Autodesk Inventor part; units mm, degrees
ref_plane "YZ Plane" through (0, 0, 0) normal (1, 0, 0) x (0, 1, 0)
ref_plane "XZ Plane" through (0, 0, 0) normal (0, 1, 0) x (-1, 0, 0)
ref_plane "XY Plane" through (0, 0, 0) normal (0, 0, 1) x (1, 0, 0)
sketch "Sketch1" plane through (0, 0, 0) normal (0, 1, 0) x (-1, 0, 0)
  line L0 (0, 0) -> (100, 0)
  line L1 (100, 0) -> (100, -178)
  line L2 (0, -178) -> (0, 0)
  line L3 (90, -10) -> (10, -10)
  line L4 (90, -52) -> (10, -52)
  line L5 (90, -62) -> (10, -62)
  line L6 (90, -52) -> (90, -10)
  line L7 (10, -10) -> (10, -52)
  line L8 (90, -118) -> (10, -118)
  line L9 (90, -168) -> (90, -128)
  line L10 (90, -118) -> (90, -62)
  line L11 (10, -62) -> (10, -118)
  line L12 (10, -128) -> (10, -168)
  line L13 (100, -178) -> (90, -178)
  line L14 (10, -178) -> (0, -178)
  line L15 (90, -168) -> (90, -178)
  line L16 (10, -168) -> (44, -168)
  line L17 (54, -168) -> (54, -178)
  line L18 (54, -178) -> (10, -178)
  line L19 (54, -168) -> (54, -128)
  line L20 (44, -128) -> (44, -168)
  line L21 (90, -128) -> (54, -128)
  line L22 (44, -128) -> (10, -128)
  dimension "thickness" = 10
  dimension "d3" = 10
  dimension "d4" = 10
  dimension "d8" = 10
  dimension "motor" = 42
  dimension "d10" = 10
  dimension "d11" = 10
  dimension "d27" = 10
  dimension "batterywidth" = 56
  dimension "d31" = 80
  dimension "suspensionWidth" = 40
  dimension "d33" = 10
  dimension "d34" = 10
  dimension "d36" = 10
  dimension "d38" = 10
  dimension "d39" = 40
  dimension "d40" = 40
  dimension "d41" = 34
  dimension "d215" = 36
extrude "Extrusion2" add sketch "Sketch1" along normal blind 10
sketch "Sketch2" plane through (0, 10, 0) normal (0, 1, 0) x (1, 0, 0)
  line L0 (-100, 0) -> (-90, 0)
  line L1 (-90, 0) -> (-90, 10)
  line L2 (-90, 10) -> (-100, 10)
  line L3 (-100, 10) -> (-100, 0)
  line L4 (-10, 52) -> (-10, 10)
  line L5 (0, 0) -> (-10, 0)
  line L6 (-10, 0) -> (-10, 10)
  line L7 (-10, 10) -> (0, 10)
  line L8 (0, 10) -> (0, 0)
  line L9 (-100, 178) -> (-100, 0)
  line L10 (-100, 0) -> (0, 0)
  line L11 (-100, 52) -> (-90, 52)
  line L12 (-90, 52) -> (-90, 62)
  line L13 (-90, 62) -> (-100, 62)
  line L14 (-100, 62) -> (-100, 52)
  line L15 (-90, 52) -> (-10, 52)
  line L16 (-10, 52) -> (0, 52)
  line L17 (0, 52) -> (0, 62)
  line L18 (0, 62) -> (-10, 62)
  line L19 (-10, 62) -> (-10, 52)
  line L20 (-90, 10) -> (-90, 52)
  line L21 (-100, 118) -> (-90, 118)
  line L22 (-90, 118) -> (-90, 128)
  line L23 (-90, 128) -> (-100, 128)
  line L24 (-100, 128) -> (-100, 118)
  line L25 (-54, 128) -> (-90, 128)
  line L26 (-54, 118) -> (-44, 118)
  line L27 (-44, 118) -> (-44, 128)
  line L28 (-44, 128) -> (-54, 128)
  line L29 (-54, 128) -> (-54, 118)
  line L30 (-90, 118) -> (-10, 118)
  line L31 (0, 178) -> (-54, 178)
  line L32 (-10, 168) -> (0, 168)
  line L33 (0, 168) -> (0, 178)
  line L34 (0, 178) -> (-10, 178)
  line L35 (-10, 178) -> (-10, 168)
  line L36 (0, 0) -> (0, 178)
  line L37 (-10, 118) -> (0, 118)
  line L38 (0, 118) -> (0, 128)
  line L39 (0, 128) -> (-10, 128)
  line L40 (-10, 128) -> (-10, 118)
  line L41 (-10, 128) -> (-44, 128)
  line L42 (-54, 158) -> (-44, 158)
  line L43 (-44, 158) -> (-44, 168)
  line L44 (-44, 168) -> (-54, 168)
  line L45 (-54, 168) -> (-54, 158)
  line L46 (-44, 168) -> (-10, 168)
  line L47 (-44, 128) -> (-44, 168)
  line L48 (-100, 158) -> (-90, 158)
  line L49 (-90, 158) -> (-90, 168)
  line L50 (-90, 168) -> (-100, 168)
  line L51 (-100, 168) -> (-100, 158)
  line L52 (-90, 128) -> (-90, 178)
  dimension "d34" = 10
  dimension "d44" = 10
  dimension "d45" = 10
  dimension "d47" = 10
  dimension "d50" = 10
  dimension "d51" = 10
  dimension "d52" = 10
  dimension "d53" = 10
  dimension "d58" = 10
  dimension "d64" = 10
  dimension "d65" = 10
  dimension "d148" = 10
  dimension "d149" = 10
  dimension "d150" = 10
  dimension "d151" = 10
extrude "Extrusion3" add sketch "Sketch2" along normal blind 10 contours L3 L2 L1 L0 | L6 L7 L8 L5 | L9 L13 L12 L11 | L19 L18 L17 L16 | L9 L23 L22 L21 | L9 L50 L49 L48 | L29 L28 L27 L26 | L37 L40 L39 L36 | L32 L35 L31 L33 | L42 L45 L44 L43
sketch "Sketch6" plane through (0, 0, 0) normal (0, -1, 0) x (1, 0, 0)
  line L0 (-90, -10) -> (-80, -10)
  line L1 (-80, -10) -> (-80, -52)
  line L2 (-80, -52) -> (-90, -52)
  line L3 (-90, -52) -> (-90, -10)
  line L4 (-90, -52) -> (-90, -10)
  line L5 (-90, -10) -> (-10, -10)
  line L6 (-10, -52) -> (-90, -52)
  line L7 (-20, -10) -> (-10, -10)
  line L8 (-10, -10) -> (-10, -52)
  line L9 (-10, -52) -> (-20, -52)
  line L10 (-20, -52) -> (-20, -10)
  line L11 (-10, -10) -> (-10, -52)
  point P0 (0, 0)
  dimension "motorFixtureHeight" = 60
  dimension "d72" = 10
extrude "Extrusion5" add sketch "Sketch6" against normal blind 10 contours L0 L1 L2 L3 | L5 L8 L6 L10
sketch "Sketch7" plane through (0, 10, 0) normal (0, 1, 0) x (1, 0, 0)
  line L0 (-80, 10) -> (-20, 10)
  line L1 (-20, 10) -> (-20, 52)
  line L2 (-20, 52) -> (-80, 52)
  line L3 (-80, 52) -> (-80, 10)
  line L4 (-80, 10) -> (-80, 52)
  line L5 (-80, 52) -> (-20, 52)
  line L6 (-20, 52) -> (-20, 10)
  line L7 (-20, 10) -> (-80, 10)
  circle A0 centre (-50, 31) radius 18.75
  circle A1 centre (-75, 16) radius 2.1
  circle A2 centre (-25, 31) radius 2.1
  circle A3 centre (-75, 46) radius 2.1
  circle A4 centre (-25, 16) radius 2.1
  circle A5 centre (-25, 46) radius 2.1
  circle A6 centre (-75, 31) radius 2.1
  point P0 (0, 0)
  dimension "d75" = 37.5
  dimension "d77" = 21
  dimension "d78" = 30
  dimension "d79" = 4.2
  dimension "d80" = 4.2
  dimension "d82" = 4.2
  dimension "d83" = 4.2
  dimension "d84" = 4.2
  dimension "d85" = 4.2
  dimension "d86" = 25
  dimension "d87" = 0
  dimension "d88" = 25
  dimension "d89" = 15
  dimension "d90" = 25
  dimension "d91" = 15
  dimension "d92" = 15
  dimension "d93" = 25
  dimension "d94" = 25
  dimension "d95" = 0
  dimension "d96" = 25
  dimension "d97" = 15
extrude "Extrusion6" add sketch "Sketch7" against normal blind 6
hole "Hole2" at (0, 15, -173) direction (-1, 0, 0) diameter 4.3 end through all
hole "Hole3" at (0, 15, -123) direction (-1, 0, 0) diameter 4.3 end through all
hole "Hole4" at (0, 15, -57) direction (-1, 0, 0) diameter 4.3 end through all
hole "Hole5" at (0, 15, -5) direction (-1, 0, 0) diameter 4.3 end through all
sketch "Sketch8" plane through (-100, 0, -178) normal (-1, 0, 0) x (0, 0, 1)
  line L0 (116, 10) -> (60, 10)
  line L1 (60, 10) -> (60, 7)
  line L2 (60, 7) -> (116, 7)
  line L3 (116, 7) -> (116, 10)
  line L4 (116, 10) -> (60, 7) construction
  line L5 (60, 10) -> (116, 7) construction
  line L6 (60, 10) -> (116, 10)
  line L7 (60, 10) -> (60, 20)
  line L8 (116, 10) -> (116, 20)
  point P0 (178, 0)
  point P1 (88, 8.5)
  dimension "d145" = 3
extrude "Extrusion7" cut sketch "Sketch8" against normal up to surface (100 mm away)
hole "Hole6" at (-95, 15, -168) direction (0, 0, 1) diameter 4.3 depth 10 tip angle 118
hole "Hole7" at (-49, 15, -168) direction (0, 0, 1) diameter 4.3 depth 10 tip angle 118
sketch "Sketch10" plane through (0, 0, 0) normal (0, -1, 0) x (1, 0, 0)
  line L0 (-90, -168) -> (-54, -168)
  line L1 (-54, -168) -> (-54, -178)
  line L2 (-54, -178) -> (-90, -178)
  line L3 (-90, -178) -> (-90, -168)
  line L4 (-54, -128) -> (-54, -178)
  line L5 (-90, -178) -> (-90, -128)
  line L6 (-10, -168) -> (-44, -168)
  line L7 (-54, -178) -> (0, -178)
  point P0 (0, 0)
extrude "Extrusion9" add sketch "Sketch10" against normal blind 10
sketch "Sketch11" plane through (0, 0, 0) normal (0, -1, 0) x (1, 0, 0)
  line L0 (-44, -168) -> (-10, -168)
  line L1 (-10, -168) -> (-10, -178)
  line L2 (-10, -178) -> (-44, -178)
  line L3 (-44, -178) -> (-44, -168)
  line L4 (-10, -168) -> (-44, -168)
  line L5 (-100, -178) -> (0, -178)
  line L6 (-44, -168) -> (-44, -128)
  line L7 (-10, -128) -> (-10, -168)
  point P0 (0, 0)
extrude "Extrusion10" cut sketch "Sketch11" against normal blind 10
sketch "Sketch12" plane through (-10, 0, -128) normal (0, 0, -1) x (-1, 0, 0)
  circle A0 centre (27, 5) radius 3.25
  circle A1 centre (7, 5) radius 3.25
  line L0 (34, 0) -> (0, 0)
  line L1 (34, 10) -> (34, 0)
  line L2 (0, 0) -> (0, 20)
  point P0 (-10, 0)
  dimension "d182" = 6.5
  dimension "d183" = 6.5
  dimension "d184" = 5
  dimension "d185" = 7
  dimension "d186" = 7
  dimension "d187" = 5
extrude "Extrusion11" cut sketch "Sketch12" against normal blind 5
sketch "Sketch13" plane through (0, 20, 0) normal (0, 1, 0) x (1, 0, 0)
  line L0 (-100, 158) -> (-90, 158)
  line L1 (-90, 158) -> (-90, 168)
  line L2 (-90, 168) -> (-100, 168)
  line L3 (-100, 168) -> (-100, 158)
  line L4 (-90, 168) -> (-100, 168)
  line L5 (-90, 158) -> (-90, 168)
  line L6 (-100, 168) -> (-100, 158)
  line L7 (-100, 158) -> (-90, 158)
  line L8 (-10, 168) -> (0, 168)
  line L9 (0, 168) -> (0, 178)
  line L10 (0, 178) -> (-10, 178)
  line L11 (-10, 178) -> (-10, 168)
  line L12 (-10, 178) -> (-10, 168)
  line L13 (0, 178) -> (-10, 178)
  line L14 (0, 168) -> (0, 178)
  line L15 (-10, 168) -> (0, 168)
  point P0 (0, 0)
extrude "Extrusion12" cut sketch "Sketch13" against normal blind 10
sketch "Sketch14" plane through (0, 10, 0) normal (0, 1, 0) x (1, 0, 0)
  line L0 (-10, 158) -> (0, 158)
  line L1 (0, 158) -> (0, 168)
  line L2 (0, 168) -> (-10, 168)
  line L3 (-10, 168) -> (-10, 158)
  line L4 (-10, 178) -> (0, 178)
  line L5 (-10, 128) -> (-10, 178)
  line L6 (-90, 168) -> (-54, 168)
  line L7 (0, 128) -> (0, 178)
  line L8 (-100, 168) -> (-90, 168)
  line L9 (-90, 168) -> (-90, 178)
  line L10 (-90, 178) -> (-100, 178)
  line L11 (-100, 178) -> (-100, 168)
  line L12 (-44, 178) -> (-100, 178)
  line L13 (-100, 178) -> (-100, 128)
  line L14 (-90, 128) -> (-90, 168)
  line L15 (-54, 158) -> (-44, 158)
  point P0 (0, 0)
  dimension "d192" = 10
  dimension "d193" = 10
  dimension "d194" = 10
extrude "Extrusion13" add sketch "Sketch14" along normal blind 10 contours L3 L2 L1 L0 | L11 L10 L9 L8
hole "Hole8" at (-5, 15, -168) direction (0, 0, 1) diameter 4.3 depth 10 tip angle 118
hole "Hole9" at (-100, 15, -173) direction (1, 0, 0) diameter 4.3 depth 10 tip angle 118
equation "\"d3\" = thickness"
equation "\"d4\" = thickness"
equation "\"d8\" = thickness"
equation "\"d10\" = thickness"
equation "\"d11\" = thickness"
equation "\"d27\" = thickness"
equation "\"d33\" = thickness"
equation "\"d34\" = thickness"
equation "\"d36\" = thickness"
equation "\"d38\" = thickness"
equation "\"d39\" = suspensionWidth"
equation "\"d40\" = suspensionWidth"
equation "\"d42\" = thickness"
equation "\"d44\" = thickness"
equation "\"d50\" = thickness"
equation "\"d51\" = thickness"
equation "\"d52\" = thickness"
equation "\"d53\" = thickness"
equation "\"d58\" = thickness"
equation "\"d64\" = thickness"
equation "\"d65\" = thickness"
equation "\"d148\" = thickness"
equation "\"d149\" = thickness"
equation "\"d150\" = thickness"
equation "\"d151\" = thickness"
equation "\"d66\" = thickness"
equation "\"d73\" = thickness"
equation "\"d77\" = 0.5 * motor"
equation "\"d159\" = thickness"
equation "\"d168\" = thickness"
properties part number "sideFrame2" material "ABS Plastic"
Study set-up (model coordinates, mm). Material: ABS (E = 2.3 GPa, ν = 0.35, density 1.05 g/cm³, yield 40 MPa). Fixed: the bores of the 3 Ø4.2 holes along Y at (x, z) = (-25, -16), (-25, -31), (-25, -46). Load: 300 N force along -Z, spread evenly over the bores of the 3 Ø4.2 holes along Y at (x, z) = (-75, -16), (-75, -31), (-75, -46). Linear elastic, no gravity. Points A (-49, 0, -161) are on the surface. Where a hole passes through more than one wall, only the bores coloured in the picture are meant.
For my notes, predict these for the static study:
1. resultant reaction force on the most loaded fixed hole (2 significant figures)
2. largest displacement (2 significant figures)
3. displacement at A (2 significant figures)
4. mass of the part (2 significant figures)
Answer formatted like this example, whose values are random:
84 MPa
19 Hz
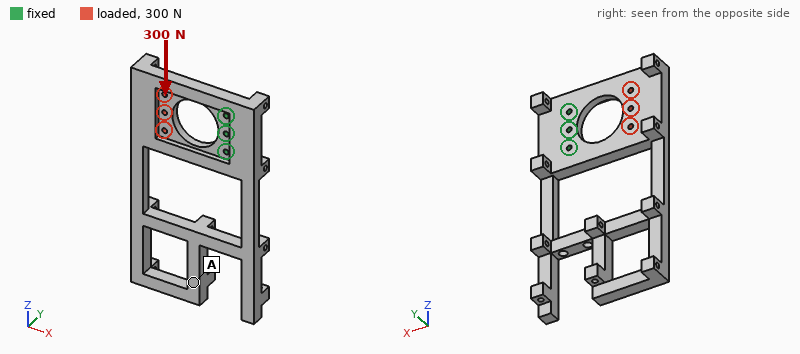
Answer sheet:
440 N
0.91 mm
0.66 mm
94 g
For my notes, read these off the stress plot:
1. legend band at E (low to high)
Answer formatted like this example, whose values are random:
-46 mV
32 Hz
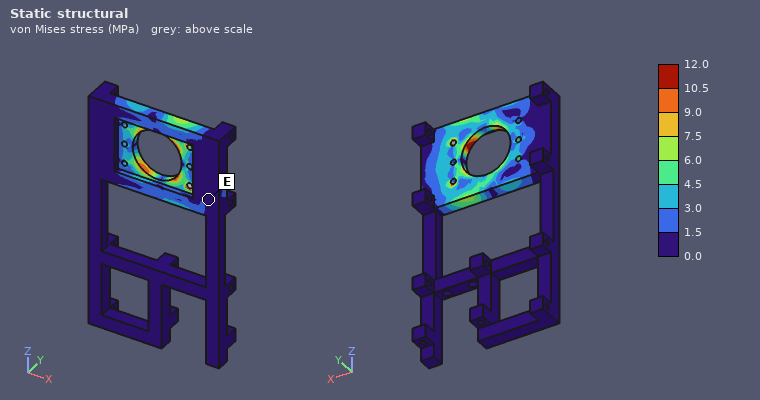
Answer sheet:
0.0 to 1.5 MPa
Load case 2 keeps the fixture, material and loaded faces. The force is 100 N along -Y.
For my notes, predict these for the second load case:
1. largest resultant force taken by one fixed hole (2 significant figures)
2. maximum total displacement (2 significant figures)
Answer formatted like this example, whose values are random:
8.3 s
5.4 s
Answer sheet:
80 N
2.2 mm
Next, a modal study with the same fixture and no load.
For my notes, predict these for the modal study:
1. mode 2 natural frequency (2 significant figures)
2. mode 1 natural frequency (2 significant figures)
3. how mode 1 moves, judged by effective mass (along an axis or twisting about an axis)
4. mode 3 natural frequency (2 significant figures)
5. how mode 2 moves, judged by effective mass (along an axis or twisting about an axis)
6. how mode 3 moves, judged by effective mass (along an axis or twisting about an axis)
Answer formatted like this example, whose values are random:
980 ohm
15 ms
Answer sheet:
140 Hz
54 Hz
along Y
200 Hz
twisting about Z
along X
